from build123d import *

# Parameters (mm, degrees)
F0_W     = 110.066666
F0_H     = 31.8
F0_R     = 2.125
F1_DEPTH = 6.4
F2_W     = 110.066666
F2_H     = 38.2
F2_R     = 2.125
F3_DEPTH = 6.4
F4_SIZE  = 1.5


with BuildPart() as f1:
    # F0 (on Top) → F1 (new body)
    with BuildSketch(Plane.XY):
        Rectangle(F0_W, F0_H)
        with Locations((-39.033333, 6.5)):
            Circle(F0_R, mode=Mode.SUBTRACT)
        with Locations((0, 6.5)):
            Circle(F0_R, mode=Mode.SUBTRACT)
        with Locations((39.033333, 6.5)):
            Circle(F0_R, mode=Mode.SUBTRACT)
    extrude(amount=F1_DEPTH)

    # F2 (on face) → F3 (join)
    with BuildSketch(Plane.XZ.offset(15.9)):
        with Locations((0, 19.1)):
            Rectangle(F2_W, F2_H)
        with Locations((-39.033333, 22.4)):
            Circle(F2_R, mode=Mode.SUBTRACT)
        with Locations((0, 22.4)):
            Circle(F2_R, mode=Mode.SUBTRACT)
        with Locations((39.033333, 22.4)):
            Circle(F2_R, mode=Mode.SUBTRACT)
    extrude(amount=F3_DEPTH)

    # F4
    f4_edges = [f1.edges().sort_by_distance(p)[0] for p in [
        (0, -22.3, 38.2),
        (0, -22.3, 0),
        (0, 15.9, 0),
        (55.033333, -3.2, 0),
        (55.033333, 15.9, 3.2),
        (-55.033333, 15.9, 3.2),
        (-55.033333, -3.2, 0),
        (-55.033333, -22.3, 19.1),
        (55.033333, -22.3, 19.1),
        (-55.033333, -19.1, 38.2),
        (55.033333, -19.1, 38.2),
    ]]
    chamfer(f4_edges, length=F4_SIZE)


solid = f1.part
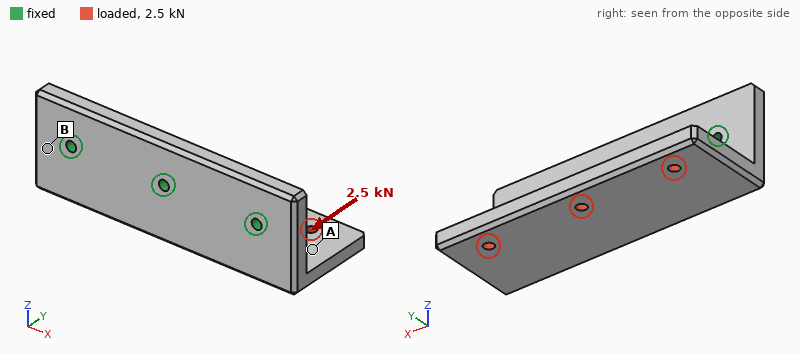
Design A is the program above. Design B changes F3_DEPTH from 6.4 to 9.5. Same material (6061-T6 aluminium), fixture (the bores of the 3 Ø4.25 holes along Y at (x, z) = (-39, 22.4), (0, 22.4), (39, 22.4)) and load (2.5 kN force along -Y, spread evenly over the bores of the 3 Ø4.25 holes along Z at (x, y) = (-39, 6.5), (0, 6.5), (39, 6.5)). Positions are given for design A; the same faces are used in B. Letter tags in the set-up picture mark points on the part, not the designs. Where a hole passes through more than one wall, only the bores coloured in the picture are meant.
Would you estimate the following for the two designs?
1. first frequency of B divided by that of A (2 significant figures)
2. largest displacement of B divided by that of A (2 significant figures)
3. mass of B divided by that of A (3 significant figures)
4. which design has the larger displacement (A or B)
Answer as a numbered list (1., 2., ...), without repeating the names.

1. 1.4
2. 0.38
3. 1.27
4. A
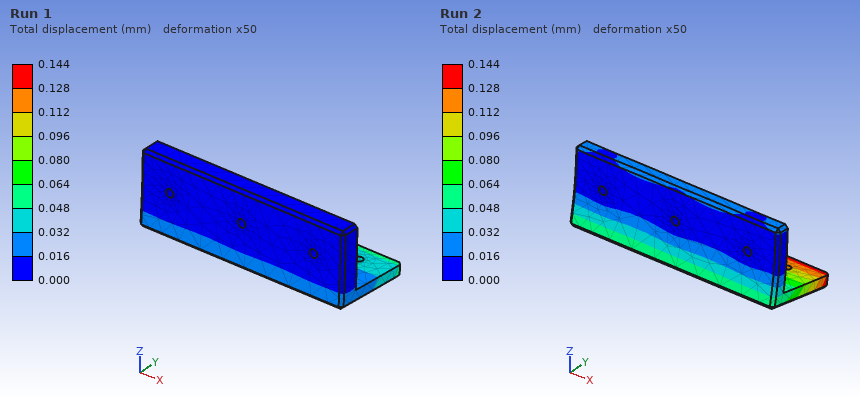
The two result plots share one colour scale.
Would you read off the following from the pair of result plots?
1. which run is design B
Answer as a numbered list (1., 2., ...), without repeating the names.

1. Run 1
